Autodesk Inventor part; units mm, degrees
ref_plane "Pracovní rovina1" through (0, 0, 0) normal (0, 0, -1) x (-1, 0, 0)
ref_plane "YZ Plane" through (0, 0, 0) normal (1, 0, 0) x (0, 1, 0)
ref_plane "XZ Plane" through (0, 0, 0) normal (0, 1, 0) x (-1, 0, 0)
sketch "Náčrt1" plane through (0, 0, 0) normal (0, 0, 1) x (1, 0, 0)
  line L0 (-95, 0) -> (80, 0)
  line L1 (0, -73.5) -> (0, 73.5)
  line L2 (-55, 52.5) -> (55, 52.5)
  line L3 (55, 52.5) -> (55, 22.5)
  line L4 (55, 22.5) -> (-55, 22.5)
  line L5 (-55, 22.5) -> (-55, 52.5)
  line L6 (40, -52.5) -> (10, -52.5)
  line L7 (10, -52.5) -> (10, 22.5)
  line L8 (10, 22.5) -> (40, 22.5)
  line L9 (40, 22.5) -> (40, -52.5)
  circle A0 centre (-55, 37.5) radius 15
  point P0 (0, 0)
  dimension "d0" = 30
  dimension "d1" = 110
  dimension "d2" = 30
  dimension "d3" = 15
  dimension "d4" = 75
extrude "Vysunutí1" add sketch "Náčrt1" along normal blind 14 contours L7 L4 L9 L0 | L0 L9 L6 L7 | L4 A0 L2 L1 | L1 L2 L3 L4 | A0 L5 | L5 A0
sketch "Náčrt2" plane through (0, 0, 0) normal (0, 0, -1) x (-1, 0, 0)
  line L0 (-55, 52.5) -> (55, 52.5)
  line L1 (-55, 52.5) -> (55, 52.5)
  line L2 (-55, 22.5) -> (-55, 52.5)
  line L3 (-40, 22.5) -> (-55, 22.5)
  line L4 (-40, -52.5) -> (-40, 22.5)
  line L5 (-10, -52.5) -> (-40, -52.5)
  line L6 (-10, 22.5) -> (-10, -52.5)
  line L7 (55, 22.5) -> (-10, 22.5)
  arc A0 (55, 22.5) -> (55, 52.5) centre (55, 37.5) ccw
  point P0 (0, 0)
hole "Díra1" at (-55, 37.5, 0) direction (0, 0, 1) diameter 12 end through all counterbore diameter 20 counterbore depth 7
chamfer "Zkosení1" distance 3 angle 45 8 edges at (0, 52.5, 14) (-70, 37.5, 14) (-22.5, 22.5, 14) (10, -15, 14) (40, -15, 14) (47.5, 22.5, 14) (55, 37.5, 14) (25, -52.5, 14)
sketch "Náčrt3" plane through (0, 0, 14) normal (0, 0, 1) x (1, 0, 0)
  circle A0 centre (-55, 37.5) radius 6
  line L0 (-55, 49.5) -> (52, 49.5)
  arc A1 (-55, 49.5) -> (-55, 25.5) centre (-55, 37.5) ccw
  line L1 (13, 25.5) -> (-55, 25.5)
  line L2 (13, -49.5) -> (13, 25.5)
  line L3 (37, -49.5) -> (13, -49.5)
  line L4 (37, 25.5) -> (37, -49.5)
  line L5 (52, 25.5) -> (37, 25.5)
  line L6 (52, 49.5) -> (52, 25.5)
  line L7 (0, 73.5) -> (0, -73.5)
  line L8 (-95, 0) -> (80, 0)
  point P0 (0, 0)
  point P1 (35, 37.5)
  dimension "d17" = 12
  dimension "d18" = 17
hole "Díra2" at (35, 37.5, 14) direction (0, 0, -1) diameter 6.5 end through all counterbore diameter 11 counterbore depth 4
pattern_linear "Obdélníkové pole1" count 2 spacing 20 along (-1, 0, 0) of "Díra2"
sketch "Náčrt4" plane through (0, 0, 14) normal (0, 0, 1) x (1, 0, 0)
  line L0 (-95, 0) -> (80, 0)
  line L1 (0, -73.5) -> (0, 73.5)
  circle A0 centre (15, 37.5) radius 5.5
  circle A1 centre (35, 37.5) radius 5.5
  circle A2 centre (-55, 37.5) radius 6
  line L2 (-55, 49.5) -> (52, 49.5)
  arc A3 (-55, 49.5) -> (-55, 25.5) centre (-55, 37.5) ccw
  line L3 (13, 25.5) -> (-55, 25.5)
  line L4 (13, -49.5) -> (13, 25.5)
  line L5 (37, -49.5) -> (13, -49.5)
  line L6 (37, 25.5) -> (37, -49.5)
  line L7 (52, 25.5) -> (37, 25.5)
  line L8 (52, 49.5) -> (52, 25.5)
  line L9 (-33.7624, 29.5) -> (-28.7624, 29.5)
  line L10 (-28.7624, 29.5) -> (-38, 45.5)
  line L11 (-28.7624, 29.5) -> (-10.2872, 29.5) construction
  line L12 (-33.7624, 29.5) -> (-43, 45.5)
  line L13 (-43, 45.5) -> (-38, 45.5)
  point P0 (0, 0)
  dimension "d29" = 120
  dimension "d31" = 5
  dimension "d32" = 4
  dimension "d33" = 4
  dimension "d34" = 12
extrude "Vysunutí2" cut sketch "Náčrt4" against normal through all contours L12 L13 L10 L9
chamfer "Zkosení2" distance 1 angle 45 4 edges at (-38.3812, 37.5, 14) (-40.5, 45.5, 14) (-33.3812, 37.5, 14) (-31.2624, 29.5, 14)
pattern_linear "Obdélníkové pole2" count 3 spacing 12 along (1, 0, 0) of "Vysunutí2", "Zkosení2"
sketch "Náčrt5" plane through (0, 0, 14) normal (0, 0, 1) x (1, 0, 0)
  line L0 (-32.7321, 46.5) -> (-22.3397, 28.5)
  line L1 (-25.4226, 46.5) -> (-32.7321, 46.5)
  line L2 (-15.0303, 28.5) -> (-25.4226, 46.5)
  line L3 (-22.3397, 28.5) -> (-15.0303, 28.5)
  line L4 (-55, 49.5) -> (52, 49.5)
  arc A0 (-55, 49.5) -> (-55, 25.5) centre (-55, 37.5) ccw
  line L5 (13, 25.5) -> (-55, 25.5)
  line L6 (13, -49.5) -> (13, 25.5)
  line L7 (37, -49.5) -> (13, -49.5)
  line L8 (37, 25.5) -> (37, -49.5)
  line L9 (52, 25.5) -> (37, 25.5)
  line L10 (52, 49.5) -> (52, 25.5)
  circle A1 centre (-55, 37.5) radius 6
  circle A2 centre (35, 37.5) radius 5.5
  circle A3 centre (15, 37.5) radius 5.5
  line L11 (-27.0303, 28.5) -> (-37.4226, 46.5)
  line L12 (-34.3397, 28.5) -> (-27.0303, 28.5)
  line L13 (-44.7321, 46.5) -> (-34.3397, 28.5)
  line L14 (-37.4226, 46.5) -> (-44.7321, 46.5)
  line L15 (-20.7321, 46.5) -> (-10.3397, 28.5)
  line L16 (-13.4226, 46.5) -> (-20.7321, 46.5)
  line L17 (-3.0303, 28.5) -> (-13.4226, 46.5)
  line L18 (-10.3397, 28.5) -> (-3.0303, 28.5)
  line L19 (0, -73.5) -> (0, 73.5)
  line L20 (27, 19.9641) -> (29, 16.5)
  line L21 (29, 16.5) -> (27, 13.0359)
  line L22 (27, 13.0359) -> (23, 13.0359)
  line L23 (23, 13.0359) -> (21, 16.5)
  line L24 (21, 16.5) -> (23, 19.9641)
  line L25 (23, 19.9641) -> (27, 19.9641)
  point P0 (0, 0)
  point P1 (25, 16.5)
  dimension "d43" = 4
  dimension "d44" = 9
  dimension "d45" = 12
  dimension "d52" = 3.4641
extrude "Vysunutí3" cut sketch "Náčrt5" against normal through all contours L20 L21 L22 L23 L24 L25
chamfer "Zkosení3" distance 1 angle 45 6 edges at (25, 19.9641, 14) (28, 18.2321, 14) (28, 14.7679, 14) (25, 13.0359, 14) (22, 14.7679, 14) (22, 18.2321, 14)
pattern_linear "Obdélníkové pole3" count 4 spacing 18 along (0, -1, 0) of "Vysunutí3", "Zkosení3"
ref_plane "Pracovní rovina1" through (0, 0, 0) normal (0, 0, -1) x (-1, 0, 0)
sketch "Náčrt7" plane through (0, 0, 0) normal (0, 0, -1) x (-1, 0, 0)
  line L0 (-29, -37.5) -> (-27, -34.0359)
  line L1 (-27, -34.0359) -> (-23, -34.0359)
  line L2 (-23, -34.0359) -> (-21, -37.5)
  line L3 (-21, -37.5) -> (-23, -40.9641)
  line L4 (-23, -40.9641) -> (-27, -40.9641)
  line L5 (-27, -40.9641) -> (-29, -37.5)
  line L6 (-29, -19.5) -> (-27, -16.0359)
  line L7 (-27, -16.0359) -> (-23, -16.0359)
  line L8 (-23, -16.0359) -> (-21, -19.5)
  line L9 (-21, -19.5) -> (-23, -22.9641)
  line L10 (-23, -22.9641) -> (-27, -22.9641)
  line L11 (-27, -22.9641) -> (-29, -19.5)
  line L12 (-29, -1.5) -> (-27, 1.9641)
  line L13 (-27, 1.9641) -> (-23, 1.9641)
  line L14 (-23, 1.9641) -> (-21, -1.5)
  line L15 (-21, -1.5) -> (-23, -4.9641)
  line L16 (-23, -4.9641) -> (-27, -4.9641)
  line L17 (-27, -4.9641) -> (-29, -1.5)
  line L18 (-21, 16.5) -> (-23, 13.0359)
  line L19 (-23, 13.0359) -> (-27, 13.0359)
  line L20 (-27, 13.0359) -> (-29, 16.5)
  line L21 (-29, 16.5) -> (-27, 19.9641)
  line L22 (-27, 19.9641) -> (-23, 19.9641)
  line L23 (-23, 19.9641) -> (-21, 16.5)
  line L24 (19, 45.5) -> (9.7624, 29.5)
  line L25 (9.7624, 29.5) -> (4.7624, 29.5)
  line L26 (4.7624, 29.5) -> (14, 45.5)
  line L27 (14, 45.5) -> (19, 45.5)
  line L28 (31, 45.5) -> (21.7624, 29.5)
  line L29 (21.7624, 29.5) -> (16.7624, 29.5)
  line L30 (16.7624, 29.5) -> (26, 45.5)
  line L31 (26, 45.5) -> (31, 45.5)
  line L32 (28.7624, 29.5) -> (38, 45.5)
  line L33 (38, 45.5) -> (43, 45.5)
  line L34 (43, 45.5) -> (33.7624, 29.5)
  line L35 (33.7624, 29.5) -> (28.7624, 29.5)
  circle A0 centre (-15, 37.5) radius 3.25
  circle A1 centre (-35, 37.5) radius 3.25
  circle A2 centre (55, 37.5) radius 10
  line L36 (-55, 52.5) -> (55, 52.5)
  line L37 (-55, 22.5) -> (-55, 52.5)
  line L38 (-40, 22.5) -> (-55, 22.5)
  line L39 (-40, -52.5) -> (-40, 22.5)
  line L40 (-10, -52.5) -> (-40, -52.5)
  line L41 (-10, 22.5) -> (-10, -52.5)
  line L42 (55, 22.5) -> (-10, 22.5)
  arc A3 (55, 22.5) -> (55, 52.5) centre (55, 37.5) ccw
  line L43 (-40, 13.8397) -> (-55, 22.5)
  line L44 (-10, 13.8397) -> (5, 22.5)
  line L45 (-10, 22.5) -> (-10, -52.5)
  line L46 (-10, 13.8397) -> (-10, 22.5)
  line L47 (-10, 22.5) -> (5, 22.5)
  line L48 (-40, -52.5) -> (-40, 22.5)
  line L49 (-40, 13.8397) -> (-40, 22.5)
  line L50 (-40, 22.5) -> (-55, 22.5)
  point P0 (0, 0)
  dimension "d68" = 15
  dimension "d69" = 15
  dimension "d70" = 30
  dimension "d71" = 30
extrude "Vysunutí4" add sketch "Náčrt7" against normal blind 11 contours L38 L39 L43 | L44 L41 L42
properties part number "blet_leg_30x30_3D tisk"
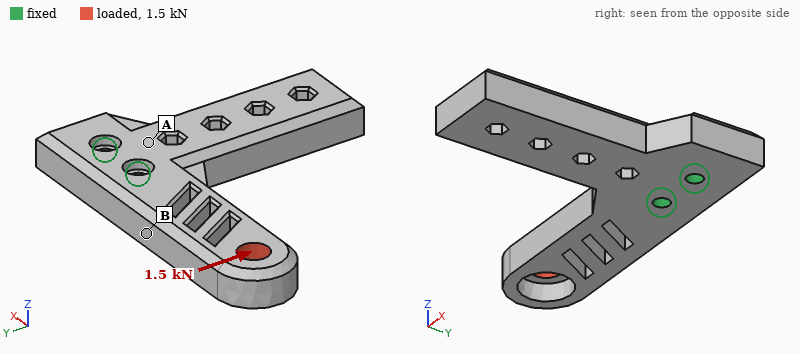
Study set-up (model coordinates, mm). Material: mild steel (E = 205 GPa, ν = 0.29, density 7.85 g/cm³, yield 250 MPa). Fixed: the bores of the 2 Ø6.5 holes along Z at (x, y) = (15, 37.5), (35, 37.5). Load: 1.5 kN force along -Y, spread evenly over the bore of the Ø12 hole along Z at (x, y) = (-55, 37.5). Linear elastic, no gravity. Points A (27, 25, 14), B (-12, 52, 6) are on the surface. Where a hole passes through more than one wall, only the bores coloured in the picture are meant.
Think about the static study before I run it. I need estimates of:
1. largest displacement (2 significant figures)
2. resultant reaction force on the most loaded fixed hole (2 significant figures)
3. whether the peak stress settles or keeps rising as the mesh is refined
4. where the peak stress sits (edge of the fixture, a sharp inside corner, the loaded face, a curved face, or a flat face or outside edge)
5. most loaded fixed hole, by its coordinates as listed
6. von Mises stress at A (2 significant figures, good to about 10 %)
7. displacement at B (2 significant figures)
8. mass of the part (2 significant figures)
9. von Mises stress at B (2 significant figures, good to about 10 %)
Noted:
67 µm
5.2 kN
keeps rising
edge of the fixture
(15, 37.5)
13 MPa
14 µm
560 g
53 MPa
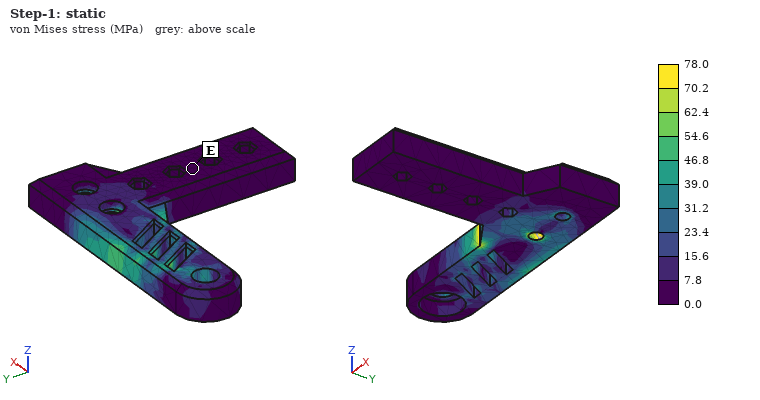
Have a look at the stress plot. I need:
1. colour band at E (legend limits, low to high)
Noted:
0.0 to 7.8 MPa
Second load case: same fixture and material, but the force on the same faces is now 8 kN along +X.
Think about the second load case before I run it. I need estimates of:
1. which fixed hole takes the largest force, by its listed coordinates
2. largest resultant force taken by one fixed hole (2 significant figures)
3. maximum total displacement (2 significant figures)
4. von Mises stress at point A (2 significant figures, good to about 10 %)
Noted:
(15, 37.5)
5.7 kN
0.14 mm
13 MPa
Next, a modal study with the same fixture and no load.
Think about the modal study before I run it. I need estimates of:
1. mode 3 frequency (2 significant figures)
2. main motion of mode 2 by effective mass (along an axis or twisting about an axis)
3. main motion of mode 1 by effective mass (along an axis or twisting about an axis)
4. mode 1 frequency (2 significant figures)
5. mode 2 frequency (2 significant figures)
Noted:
2800 Hz
along Z
along Z
1400 Hz
1600 Hz
